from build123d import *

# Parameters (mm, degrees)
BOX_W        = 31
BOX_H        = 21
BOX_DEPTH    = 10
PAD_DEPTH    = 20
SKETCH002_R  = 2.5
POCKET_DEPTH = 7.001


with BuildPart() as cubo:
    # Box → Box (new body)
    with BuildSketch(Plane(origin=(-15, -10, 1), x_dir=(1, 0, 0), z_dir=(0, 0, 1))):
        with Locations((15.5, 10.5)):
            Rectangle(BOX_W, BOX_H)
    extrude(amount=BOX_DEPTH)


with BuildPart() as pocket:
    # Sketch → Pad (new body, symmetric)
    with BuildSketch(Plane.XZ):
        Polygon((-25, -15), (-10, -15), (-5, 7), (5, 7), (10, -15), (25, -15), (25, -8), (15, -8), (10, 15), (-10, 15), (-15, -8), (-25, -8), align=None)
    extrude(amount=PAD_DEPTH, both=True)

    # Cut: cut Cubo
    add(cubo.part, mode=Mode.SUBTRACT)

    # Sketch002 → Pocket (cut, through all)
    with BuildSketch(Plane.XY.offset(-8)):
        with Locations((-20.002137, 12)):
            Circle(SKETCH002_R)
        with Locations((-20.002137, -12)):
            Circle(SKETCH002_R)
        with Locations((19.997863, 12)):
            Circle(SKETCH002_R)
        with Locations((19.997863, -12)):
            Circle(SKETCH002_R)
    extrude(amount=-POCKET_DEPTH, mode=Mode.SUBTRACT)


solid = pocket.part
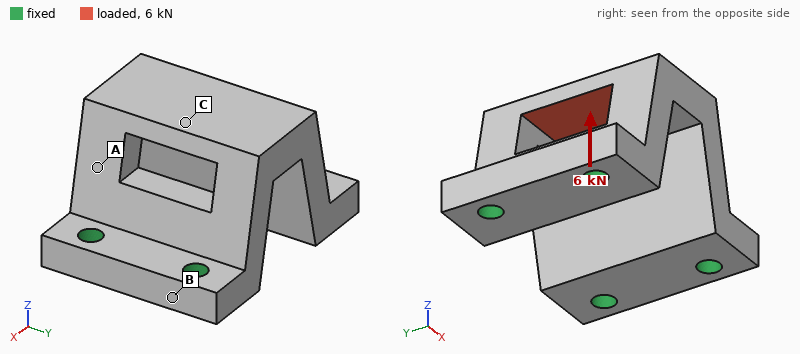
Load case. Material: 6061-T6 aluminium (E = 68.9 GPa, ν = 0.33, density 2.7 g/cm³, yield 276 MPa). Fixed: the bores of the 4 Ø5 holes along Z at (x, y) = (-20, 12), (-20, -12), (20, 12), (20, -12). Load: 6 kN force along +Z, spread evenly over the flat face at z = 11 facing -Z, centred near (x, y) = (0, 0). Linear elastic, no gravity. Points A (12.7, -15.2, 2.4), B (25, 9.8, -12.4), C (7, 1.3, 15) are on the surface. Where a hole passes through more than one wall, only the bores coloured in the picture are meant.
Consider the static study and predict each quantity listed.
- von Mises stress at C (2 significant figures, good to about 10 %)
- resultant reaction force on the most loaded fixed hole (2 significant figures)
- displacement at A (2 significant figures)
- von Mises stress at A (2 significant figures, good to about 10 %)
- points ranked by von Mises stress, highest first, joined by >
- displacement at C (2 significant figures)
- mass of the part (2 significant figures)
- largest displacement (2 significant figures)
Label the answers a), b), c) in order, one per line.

a) 160 MPa
b) 1.7 kN
c) 13 µm
d) 34 MPa
e) C > A > B
f) 74 µm
g) 53 g
h) 82 µm
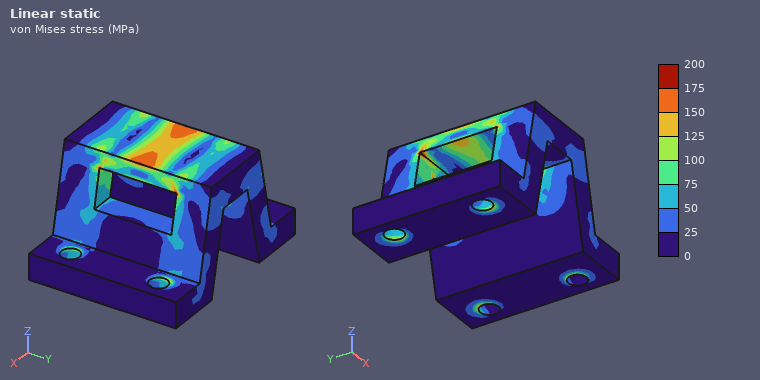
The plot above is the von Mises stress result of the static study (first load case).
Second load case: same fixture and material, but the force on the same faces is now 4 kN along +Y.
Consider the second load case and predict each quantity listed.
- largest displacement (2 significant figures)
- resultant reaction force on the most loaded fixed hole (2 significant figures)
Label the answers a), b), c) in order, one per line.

a) 81 µm
b) 2.1 kN
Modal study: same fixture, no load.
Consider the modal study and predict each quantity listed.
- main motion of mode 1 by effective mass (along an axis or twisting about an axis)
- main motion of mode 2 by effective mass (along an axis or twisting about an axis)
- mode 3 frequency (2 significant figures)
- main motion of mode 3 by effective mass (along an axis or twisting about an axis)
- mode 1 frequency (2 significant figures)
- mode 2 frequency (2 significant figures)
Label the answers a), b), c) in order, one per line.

a) along Y
b) along X
c) 14 kHz
d) twisting about Z
e) 10 kHz
f) 11 kHz
